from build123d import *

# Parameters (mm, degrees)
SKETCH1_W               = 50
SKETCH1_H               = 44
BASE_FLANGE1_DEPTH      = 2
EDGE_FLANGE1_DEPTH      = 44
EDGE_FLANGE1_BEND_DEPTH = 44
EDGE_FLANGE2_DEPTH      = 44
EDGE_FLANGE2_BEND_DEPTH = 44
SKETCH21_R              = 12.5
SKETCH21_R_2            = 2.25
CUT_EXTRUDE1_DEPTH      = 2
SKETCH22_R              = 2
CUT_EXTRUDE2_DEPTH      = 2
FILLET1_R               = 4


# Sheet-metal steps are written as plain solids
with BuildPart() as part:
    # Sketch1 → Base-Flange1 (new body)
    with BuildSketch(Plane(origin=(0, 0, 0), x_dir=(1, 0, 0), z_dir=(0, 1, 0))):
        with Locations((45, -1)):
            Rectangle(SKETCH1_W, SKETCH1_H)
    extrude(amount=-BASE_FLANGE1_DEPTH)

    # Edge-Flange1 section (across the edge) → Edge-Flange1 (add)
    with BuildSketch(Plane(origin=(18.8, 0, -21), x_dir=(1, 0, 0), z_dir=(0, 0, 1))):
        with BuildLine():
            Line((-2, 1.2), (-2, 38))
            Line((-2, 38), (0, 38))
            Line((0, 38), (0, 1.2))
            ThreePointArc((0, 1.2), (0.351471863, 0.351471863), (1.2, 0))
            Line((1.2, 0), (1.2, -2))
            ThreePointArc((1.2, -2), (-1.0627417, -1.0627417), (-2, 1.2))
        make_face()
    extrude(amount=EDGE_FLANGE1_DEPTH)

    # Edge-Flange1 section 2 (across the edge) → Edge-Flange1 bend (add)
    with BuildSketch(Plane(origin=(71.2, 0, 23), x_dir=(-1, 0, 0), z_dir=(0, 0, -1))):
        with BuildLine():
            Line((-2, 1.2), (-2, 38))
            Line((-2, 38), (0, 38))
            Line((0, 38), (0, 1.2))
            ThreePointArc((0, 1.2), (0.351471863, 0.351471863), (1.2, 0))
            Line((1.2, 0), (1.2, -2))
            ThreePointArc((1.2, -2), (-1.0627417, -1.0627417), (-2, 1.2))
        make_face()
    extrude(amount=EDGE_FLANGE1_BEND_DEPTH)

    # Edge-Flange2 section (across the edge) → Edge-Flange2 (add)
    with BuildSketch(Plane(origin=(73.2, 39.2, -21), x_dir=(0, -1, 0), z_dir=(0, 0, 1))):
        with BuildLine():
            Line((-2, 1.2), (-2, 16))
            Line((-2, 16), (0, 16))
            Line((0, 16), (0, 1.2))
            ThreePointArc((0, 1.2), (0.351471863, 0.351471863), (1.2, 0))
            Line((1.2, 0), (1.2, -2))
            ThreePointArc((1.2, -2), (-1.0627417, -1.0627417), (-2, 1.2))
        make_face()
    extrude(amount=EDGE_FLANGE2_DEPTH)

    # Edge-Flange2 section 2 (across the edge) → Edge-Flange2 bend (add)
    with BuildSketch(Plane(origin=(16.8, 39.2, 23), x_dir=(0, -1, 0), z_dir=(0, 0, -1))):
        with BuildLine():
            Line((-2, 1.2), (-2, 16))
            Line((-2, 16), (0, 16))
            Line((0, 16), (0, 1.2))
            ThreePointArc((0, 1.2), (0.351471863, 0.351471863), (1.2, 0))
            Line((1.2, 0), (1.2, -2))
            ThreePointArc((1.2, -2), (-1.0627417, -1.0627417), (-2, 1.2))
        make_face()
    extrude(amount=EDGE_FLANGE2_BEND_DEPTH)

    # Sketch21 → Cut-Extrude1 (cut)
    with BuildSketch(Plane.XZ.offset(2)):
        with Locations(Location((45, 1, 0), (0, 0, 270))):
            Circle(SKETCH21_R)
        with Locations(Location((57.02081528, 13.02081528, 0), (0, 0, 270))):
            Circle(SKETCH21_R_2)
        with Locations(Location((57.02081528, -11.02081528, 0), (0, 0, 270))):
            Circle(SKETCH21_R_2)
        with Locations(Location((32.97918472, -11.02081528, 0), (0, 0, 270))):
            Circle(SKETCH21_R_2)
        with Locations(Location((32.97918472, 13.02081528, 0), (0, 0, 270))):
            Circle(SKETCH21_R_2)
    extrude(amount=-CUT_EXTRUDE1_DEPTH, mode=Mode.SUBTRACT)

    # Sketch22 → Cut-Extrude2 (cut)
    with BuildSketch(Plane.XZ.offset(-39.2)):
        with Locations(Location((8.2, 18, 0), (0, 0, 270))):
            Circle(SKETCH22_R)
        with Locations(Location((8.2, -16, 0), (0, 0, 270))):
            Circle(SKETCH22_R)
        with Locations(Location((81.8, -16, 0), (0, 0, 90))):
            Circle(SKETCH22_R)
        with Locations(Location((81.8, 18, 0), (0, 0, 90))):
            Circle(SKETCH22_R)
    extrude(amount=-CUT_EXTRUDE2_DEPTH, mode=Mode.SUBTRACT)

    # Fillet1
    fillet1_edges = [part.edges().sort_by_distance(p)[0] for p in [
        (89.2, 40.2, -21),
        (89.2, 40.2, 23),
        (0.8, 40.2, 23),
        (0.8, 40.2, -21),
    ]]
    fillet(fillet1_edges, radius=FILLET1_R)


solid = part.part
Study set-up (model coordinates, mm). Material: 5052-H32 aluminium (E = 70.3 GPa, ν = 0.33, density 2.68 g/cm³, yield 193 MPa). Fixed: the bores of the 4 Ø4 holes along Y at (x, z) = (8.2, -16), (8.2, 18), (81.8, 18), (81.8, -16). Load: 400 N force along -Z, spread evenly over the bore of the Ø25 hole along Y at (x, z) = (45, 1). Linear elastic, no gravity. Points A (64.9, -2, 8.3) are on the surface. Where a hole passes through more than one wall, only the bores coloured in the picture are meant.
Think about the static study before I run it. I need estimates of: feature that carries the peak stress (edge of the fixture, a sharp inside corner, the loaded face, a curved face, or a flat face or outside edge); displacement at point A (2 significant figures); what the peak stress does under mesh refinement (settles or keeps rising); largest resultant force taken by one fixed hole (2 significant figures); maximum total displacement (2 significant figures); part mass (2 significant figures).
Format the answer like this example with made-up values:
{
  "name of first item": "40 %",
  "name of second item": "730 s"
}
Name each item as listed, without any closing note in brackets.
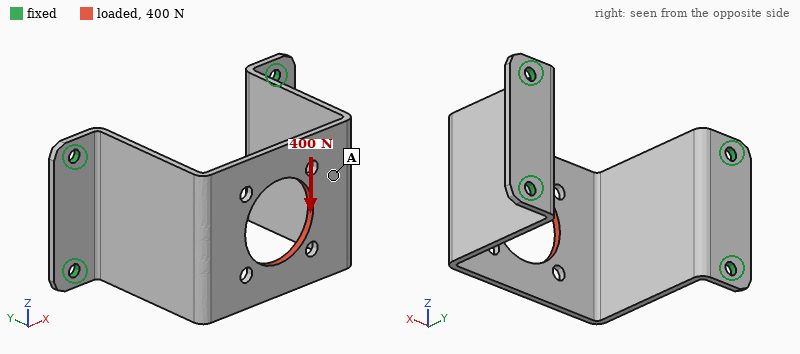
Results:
{
  "feature that carries the peak stress": "edge of the fixture",
  "displacement at point A": "0.12 mm",
  "what the peak stress does under mesh refinement": "keeps rising",
  "largest resultant force taken by one fixed hole": "270 N",
  "maximum total displacement": "0.13 mm",
  "part mass": "36 g"
}
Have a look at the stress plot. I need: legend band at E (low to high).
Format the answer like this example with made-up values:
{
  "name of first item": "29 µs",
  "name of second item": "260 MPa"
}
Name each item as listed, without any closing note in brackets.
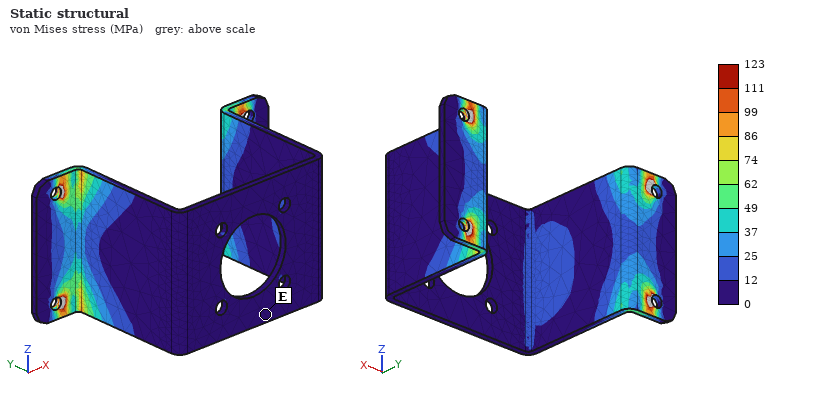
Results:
{
  "legend band at E": "0 to 12 MPa"
}
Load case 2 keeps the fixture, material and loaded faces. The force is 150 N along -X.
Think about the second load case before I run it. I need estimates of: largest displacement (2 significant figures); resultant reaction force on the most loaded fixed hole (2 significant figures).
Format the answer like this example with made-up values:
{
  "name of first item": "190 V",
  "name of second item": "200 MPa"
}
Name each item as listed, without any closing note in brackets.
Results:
{
  "largest displacement": "0.44 mm",
  "resultant reaction force on the most loaded fixed hole": "49 N"
}
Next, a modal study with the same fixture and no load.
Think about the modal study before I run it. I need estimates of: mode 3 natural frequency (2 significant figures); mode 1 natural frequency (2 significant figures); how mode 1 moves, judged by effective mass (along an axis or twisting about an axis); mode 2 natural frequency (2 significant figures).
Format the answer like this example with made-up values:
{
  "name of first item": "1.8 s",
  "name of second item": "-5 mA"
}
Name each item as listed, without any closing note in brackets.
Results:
{
  "mode 3 natural frequency": "2100 Hz",
  "mode 1 natural frequency": "730 Hz",
  "how mode 1 moves, judged by effective mass": "along X",
  "mode 2 natural frequency": "2100 Hz"
}
